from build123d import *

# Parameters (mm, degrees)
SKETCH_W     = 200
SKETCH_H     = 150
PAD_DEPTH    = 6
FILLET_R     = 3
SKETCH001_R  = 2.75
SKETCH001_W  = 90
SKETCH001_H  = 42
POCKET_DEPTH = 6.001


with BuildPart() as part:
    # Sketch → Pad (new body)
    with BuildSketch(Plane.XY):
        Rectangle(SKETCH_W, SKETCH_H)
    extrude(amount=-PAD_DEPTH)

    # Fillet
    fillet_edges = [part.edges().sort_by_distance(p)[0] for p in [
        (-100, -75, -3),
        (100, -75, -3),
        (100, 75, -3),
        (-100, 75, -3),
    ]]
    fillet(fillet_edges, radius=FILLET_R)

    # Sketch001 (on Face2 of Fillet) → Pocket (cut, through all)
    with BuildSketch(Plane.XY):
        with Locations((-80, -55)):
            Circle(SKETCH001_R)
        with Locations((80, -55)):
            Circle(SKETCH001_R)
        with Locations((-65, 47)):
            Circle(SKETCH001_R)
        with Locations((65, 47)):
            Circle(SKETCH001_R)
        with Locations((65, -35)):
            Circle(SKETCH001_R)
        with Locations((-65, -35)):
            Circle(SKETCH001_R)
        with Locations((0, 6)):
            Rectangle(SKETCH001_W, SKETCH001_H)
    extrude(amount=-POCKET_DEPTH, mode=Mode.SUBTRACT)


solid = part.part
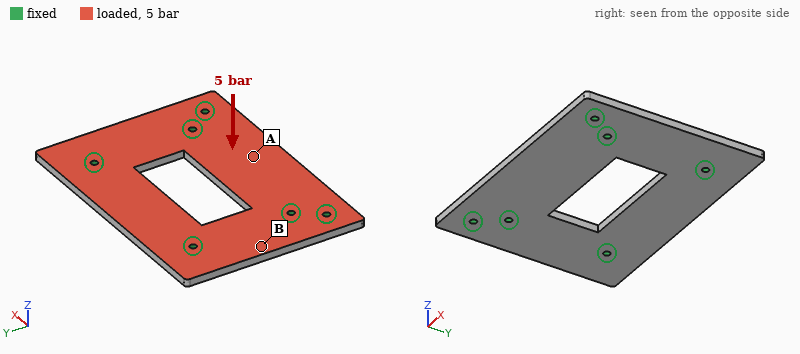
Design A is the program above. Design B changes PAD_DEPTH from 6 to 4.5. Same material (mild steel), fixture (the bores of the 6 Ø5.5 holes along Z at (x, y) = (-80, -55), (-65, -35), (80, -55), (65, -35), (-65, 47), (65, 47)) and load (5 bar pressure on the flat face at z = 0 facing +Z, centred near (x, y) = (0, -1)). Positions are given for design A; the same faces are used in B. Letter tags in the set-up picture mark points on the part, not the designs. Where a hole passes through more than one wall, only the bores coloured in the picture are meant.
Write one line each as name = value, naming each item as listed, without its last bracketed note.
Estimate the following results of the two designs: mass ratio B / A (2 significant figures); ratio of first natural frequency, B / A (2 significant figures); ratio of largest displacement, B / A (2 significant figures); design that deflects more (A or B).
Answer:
mass ratio B / A = 0.75
ratio of first natural frequency, B / A = 0.76
ratio of largest displacement, B / A = 2.3
design that deflects more = B
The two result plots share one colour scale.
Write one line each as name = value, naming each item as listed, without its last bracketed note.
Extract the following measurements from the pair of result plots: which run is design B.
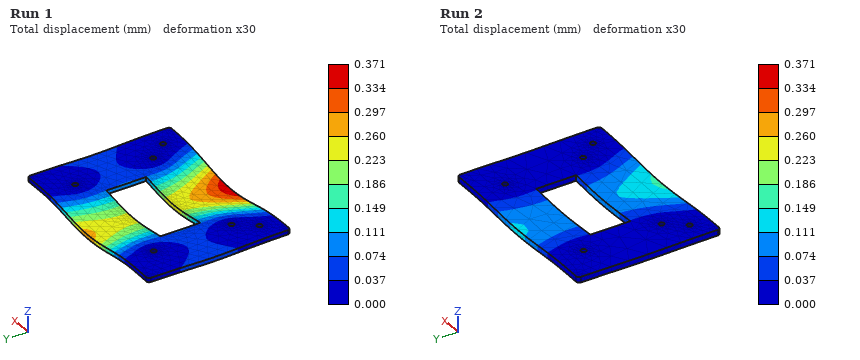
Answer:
which run is design B = Run 1
